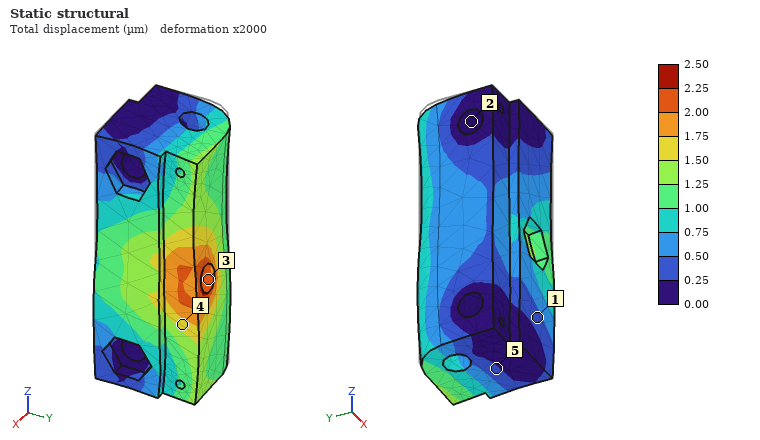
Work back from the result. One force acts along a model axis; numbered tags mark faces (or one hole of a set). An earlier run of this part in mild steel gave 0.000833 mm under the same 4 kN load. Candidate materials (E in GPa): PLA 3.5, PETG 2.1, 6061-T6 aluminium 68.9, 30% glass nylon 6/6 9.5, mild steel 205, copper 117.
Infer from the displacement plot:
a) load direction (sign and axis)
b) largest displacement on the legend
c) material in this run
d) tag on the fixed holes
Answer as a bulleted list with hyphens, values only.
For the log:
- -Z
- 2.50 µm
- 6061-T6 aluminium
- 2
